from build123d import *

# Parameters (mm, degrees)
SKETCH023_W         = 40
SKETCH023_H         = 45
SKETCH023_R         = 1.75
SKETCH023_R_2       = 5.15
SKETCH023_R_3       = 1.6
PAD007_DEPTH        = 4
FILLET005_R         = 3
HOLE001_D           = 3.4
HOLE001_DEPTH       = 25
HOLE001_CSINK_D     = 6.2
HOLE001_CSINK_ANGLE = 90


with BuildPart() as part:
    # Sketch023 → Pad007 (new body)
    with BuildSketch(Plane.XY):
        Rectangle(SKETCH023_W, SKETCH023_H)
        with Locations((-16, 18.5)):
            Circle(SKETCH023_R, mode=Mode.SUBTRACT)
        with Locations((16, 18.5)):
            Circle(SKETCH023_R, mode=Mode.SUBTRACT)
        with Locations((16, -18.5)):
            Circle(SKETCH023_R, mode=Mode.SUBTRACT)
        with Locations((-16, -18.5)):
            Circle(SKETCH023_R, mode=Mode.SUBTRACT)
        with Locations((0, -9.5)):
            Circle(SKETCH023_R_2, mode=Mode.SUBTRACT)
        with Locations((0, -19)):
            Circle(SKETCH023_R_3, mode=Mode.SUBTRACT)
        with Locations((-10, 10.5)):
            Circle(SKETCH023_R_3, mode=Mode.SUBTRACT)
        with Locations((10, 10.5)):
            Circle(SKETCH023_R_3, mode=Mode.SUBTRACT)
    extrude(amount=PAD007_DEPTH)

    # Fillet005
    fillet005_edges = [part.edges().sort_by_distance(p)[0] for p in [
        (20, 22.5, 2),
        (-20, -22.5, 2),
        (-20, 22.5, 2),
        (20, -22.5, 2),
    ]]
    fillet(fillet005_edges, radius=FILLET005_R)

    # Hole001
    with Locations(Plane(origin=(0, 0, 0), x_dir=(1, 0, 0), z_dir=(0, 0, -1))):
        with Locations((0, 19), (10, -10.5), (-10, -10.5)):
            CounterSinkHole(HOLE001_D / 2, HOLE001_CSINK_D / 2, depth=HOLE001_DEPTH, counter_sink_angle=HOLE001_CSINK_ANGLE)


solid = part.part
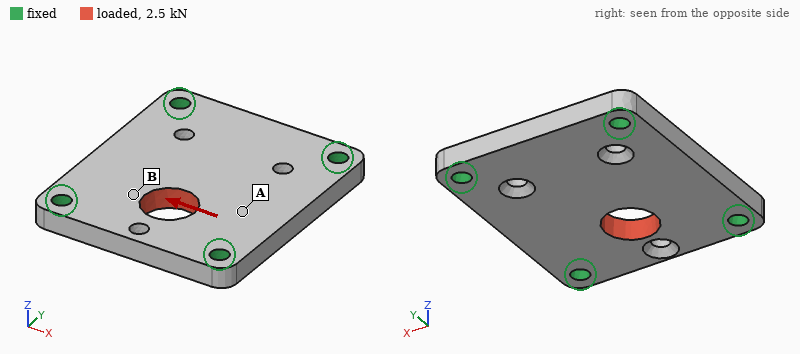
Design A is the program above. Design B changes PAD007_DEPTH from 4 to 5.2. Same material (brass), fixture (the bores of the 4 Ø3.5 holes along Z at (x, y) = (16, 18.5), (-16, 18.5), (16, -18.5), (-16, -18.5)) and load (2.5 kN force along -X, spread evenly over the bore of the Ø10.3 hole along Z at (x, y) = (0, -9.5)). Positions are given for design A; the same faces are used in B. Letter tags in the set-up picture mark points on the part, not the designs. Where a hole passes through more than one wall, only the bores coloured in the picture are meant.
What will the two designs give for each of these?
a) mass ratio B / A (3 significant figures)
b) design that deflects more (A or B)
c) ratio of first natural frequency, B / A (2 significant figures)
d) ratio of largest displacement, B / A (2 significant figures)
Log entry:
1.30
A
1.2
0.77
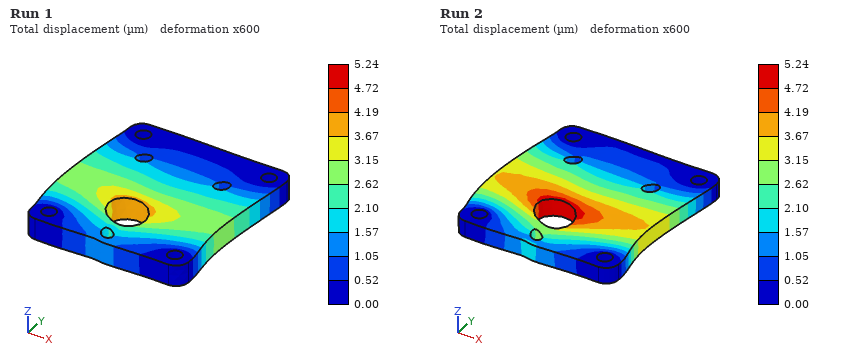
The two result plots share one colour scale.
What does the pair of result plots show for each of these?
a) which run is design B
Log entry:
Run 1
